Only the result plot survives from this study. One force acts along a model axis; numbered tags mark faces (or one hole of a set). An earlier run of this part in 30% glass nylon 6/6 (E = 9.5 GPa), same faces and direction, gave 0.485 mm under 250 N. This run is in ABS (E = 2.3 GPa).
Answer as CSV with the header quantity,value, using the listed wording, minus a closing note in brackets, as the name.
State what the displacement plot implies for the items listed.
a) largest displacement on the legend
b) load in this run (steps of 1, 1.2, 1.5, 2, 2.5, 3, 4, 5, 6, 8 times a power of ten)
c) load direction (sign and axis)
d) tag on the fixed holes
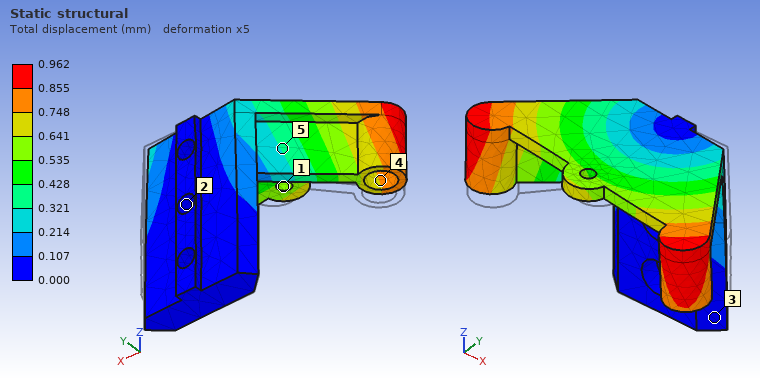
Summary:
quantity,value
largest displacement on the legend,0.962 mm
load in this run,120 N
load direction,-X
tag on the fixed holes,2
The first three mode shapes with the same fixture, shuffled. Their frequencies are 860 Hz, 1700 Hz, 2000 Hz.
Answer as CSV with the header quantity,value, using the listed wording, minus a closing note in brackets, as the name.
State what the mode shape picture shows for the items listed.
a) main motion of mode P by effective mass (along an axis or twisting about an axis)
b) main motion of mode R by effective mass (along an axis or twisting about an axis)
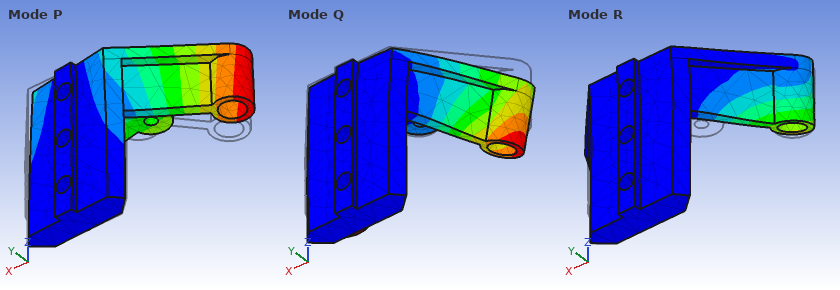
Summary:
quantity,value
main motion of mode P by effective mass,along X
main motion of mode R by effective mass,along Z
